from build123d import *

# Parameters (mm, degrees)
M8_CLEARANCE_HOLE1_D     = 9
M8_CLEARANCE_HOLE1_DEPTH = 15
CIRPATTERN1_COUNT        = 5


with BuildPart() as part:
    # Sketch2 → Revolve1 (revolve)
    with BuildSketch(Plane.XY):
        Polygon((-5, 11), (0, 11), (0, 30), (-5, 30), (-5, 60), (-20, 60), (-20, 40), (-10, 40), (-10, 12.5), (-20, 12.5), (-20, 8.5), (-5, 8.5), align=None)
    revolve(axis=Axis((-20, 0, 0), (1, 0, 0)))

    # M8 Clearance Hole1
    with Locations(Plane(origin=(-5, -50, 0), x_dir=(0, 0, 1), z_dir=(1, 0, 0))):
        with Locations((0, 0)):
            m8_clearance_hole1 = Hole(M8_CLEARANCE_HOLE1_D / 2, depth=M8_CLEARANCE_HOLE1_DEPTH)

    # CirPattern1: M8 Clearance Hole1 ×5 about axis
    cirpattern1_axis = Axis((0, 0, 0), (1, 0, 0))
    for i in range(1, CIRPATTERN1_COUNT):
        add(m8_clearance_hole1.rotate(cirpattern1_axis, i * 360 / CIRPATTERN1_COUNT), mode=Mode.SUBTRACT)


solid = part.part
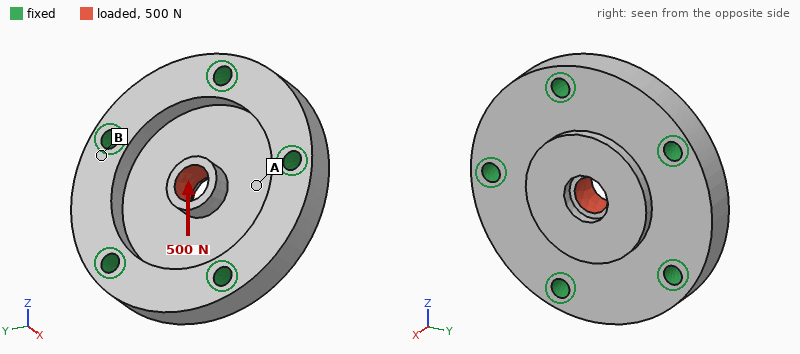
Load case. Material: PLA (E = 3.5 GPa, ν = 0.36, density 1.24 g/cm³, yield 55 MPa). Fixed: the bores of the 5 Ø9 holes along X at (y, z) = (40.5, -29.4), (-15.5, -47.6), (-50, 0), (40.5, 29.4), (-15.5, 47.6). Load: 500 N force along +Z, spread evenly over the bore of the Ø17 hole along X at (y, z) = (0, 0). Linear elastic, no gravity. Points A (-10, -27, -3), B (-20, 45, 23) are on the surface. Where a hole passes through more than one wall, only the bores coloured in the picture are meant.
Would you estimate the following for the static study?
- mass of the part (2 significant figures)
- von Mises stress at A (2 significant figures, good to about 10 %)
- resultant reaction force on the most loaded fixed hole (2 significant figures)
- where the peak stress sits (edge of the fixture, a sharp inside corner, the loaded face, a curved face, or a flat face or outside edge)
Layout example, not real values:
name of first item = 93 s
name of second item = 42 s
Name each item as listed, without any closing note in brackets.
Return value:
mass of the part = 160 g
von Mises stress at A = 0.82 MPa
resultant reaction force on the most loaded fixed hole = 120 N
where the peak stress sits = the loaded face
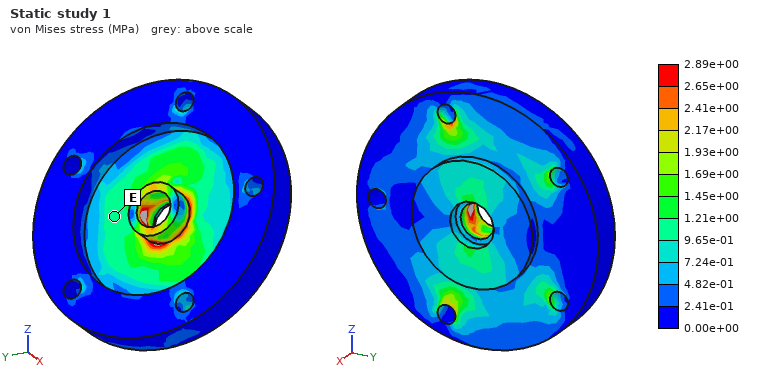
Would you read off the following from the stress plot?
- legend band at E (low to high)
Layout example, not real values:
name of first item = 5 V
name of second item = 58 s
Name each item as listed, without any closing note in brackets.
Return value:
legend band at E = 9.65e-01 to 1.21e+00 MPa
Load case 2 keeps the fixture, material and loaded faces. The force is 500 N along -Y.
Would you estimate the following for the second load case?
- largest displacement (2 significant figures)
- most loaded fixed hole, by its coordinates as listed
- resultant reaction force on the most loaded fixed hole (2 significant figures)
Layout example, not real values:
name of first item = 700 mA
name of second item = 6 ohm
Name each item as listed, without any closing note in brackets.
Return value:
largest displacement = 43 µm
most loaded fixed hole, by its coordinates as listed = (-50, 0)
resultant reaction force on the most loaded fixed hole = 130 N
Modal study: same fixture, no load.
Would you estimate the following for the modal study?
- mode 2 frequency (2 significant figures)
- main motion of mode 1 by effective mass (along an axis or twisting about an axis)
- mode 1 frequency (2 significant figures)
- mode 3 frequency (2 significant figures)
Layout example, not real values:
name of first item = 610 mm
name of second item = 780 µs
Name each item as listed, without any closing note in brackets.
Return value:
mode 2 frequency = 4400 Hz
main motion of mode 1 by effective mass = along X
mode 1 frequency = 2600 Hz
mode 3 frequency = 4400 Hz
